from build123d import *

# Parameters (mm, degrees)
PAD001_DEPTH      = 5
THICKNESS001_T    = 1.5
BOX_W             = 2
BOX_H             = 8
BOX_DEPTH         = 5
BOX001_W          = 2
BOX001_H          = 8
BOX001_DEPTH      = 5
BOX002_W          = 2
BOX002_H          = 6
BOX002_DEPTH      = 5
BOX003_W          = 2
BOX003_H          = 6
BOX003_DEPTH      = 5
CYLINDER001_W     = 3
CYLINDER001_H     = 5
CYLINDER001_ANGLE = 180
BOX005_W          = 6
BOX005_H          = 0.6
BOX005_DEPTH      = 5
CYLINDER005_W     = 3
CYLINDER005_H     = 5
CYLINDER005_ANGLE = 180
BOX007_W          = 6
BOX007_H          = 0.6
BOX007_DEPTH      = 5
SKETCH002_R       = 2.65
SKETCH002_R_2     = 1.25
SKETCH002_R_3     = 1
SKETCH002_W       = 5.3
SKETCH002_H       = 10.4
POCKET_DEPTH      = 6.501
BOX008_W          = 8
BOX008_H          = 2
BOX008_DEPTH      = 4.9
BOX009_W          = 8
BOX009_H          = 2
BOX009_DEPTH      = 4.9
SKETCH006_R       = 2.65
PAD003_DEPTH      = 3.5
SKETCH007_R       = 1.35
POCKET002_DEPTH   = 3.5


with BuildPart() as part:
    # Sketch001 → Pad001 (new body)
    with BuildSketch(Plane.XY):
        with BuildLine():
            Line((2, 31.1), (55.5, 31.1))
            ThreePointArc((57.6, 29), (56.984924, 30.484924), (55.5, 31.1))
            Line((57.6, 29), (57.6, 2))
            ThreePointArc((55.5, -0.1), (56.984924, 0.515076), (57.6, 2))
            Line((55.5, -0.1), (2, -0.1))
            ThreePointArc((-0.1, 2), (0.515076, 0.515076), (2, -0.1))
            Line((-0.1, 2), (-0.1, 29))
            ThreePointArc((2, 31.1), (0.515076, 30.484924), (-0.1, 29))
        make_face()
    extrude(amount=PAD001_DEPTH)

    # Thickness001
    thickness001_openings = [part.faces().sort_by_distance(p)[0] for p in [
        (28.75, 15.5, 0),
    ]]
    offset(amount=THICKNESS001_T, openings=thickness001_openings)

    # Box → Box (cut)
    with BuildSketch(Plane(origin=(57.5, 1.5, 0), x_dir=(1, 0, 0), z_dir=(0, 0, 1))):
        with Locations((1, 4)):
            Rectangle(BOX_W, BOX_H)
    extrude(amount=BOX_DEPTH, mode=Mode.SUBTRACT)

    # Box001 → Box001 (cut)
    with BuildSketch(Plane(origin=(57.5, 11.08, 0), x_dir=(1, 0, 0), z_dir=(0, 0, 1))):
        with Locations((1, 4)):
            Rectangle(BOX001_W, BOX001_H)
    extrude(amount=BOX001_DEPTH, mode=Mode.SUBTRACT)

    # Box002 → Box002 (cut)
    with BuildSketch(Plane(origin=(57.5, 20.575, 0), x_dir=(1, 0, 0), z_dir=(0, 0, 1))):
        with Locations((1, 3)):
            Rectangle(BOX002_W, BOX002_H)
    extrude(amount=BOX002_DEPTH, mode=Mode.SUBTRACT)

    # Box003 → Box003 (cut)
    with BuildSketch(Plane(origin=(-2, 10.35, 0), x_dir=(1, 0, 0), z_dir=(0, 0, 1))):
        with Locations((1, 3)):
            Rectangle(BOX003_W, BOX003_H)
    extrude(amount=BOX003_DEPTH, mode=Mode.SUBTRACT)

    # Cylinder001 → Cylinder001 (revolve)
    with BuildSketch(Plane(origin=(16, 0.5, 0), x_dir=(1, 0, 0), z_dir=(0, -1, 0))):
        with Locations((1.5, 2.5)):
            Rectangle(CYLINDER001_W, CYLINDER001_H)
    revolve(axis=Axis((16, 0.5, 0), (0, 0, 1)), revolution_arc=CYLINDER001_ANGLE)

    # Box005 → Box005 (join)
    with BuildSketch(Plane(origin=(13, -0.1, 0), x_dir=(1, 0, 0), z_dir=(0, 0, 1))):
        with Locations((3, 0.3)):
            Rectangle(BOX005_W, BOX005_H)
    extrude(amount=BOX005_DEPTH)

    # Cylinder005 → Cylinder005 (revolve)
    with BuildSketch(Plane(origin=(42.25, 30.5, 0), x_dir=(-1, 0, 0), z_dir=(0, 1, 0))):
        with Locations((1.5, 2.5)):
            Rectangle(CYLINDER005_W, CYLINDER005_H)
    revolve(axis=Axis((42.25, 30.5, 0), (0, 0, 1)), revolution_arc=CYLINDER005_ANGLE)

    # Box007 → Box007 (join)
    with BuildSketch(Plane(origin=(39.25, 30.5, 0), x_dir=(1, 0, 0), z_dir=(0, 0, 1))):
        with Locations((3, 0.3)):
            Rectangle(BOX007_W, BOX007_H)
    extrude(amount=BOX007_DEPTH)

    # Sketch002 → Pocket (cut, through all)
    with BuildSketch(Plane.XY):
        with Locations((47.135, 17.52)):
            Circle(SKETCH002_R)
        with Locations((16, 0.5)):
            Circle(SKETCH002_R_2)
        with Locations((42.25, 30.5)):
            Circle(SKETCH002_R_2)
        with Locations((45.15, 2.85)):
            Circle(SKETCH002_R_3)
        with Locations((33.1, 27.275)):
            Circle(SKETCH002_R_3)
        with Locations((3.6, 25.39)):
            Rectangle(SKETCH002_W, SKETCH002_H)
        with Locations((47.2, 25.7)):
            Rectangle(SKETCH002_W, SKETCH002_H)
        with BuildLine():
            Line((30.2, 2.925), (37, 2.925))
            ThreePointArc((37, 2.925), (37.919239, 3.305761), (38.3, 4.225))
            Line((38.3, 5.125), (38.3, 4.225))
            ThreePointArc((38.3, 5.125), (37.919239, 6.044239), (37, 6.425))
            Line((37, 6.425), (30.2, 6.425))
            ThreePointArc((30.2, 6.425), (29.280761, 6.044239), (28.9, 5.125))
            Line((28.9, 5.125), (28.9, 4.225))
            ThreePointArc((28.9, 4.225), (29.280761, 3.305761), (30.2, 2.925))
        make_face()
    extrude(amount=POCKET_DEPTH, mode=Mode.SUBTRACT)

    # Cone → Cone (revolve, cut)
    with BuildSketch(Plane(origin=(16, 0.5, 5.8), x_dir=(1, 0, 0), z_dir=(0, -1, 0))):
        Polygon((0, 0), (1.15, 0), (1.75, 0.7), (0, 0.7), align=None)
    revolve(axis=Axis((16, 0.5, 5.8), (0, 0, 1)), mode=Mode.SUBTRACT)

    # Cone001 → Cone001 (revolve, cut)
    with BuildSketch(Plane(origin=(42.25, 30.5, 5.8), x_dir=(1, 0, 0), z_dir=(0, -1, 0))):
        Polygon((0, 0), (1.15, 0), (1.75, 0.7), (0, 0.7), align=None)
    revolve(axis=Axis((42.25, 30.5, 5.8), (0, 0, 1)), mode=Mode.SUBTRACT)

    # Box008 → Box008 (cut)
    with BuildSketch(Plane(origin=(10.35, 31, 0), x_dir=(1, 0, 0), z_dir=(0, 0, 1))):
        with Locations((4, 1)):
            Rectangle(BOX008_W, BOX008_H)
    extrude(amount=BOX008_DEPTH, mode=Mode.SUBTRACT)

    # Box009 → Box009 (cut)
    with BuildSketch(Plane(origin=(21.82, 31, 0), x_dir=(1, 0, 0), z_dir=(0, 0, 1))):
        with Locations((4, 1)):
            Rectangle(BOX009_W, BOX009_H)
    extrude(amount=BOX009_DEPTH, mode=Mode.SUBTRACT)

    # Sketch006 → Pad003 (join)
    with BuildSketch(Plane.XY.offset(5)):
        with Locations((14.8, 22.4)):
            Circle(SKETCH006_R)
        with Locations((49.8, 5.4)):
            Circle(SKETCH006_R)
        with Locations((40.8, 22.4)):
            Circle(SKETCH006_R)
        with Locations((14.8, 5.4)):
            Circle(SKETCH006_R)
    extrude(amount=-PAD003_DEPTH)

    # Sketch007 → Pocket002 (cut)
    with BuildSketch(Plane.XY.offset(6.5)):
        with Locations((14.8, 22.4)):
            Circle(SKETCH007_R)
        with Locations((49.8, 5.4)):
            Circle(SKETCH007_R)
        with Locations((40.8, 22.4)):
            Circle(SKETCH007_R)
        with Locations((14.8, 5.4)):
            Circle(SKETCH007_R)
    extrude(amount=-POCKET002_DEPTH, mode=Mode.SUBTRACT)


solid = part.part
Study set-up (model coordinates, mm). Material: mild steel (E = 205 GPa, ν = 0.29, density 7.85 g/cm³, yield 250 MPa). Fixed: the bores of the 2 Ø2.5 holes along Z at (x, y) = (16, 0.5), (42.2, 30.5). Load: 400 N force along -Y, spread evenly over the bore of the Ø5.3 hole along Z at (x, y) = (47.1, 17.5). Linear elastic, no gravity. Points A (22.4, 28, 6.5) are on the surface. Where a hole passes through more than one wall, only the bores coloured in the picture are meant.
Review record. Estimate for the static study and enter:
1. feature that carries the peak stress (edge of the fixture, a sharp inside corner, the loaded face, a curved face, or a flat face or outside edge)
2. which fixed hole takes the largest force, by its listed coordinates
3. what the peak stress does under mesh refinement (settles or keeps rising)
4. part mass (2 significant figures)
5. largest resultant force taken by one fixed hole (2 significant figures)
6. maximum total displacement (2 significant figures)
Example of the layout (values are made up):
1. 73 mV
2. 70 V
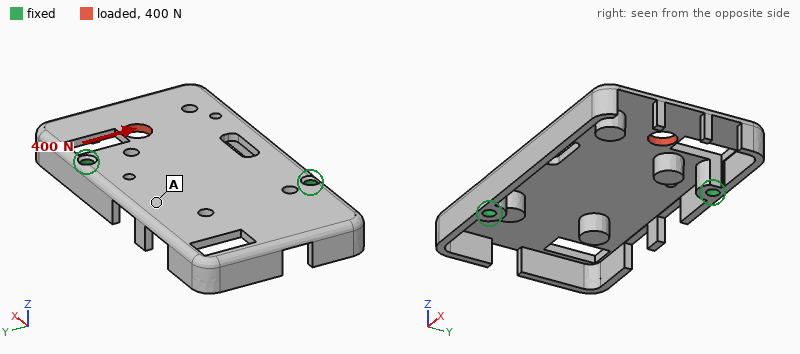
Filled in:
1. a sharp inside corner
2. (42.2, 30.5)
3. keeps rising
4. 32 g
5. 350 N
6. 11 µm
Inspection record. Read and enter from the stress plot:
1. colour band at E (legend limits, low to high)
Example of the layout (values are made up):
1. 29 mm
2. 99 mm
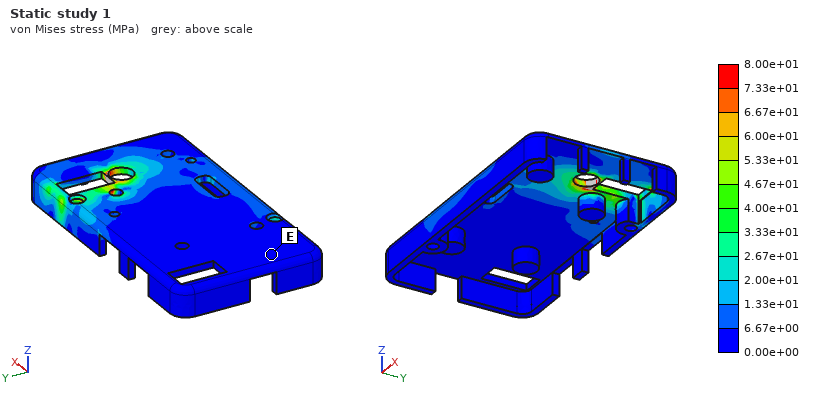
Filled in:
1. 0.00e+00 to 6.67e+00 MPa
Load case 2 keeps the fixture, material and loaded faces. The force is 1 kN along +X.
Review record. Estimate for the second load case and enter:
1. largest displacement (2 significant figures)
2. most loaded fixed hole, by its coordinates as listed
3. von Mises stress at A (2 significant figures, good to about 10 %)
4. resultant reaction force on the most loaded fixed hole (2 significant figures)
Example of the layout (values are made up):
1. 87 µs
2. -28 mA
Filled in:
1. 17 µm
2. (42.2, 30.5)
3. 11 MPa
4. 570 N
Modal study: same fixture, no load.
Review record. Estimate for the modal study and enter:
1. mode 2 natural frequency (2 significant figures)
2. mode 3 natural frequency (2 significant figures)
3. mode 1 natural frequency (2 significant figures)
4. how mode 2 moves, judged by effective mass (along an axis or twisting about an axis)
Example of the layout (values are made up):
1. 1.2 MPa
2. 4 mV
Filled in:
1. 2700 Hz
2. 5500 Hz
3. 2000 Hz
4. along Z
